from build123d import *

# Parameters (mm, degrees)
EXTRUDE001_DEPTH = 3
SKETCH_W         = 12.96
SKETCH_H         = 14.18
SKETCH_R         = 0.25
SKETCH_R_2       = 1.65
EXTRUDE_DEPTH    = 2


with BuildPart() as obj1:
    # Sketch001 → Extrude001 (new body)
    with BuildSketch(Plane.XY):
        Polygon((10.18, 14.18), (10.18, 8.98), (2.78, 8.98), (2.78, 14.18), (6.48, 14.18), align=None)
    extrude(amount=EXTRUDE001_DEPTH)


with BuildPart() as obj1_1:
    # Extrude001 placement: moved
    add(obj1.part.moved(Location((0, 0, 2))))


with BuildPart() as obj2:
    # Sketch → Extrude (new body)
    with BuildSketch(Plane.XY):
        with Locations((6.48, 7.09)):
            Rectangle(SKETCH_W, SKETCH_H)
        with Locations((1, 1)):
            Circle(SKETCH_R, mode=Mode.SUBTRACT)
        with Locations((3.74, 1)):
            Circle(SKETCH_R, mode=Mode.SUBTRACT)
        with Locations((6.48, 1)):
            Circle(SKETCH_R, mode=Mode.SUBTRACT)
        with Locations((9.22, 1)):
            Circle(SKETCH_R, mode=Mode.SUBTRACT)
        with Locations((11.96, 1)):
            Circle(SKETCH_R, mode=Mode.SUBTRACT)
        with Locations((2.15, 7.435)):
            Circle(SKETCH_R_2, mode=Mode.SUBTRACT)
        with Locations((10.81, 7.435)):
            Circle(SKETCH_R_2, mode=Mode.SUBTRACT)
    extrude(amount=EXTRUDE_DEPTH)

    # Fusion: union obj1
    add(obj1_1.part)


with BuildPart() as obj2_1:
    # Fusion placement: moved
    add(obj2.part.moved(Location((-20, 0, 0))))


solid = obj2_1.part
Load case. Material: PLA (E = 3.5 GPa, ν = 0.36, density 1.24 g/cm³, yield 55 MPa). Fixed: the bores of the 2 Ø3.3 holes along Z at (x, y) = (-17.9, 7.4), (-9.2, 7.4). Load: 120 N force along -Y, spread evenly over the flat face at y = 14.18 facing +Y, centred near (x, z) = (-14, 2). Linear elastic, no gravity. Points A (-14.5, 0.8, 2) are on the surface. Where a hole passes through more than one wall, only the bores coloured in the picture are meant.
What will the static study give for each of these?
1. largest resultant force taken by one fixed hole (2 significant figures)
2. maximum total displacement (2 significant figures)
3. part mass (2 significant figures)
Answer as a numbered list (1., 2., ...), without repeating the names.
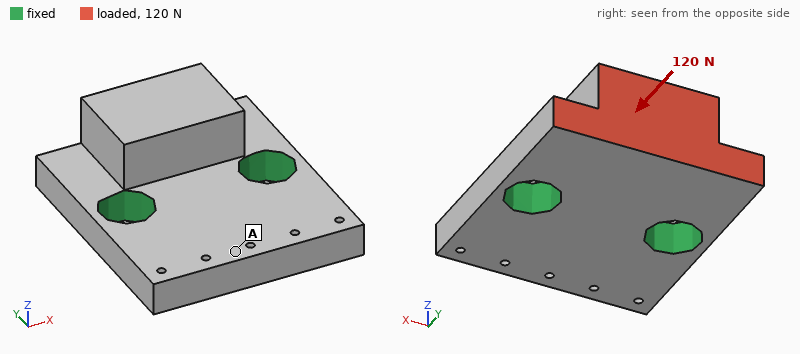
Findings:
1. 62 N
2. 54 µm
3. 0.55 g
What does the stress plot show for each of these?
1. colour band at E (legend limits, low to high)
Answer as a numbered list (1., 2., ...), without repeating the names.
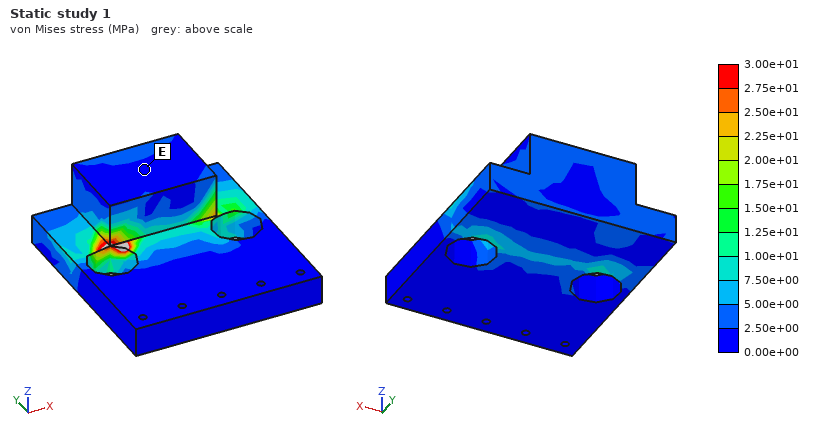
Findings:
1. 0.00e+00 to 2.50e+00 MPa
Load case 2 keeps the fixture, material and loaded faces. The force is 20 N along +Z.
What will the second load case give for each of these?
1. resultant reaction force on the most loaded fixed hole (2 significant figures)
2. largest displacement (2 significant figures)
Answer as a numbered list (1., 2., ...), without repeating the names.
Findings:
1. 10 N
2. 39 µm
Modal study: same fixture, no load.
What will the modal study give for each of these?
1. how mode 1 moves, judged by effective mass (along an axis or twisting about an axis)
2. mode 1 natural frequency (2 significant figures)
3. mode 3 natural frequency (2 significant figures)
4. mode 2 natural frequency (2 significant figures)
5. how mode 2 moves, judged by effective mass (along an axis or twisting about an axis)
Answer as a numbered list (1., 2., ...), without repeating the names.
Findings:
1. along Z
2. 11 kHz
3. 19 kHz
4. 13 kHz
5. along Z
